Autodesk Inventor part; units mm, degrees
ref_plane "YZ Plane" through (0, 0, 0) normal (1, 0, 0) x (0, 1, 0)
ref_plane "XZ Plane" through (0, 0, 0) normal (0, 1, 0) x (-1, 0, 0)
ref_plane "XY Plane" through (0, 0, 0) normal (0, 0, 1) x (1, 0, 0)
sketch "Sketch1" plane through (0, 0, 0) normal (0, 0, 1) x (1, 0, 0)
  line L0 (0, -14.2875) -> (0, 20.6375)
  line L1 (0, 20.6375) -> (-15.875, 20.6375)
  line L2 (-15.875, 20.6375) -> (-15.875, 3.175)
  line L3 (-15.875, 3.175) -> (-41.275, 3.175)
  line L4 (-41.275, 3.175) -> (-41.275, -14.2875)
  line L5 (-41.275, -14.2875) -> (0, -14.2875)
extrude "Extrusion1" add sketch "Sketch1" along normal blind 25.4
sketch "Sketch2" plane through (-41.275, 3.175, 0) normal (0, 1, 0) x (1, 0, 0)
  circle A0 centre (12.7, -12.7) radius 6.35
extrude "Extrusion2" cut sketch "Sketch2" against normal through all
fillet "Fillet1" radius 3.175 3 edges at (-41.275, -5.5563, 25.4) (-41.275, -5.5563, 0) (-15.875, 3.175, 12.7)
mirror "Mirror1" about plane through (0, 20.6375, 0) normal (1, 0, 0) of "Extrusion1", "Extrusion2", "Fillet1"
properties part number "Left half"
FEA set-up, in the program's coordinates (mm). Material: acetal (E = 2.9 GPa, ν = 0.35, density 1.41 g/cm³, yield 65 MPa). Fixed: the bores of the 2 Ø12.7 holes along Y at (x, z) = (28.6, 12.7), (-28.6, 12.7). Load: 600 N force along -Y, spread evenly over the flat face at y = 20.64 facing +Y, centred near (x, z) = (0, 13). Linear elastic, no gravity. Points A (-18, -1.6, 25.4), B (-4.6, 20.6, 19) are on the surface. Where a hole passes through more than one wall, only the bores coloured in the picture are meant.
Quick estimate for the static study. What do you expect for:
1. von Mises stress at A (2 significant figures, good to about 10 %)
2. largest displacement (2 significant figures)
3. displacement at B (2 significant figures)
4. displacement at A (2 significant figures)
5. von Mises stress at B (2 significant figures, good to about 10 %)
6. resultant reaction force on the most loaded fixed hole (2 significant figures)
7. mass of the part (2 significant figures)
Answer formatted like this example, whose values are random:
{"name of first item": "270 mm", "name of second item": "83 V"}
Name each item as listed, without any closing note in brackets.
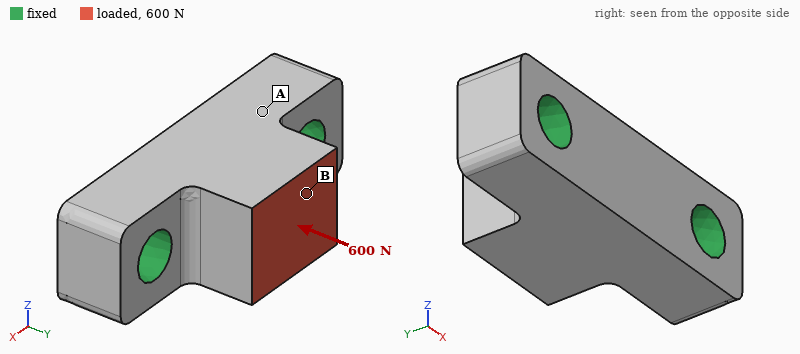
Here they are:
{"von Mises stress at A": "1.4 MPa", "largest displacement": "16 µm", "displacement at B": "16 µm", "displacement at A": "6.9 µm", "von Mises stress at B": "0.68 MPa", "resultant reaction force on the most loaded fixed hole": "320 N", "mass of the part": "65 g"}
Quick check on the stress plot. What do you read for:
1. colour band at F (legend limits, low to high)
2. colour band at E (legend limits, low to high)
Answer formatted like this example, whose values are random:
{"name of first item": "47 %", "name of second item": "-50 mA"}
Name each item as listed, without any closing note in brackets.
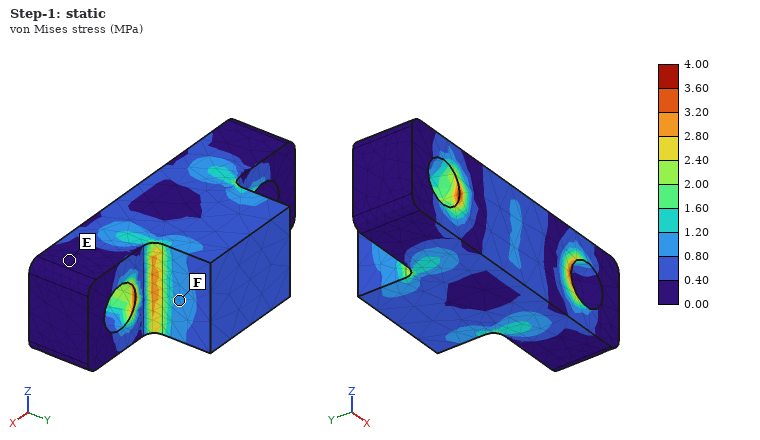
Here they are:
{"colour band at F": "0.80 to 1.20 MPa", "colour band at E": "0.00 to 0.40 MPa"}
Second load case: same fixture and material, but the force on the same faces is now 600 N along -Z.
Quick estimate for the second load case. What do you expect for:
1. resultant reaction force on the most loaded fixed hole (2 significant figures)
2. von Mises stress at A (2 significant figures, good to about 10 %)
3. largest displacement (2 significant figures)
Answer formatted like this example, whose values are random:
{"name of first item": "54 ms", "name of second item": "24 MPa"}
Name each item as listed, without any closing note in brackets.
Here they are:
{"resultant reaction force on the most loaded fixed hole": "300 N", "von Mises stress at A": "6.9 MPa", "largest displacement": "0.14 mm"}
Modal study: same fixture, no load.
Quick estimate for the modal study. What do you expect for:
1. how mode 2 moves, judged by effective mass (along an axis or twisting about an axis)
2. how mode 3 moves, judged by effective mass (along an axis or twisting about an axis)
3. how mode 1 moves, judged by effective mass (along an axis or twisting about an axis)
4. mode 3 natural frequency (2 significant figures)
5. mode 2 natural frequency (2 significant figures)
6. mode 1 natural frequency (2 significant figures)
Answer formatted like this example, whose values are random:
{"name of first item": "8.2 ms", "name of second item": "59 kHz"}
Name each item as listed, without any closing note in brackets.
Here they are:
{"how mode 2 moves, judged by effective mass": "along Y", "how mode 3 moves, judged by effective mass": "along X", "how mode 1 moves, judged by effective mass": "along Z", "mode 3 natural frequency": "6500 Hz", "mode 2 natural frequency": "5500 Hz", "mode 1 natural frequency": "3100 Hz"}
